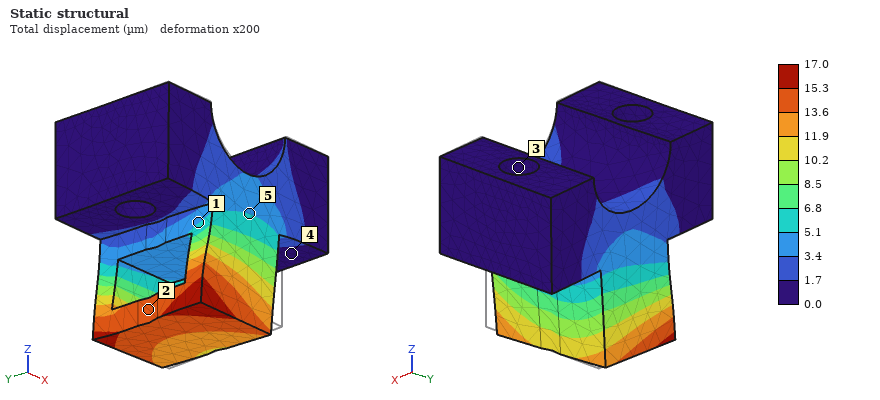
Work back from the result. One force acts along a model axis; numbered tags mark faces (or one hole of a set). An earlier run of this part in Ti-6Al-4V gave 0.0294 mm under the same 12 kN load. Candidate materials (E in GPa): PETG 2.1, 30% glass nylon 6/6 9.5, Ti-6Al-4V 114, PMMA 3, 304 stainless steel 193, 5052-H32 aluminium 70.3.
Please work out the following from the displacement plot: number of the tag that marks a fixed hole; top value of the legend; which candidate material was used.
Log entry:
3
17.0 µm
304 stainless steel
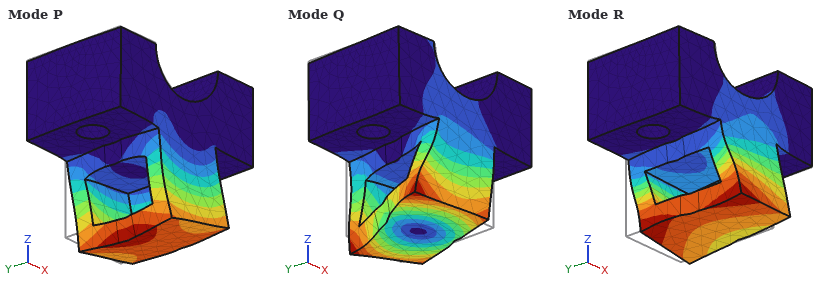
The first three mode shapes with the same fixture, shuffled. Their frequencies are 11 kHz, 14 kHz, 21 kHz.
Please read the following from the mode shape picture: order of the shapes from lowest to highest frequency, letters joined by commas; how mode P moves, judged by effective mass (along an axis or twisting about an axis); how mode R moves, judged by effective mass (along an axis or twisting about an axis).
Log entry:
R, P, Q
along X
along Y
